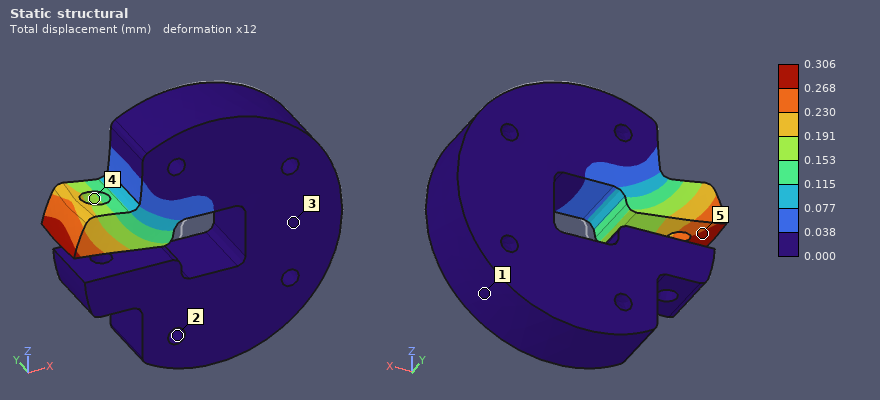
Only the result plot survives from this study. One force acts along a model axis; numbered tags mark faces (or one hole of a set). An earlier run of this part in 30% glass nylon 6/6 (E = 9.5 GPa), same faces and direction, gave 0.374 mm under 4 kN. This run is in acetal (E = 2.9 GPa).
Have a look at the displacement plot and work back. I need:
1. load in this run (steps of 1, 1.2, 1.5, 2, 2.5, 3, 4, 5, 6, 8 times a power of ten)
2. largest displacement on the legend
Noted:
1 kN
0.306 mm
